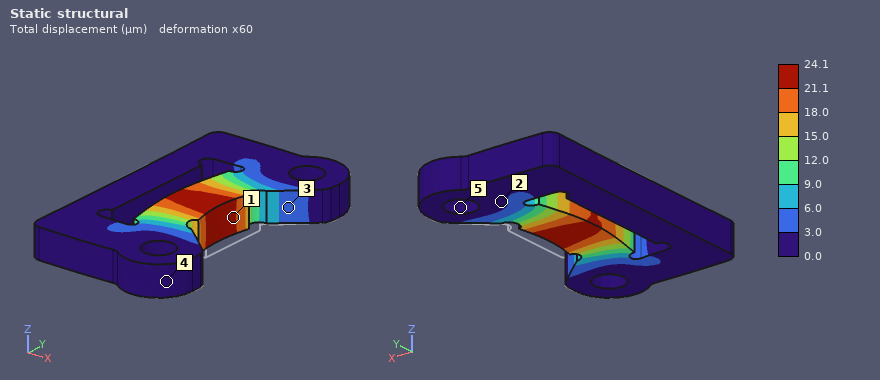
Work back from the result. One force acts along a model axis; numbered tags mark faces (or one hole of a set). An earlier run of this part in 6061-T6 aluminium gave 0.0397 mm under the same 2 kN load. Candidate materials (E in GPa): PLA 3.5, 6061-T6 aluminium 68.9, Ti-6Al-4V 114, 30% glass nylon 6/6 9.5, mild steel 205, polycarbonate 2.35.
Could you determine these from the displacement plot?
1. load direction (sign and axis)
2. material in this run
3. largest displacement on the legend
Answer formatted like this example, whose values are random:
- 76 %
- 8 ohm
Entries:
- -X
- Ti-6Al-4V
- 24.1 µm
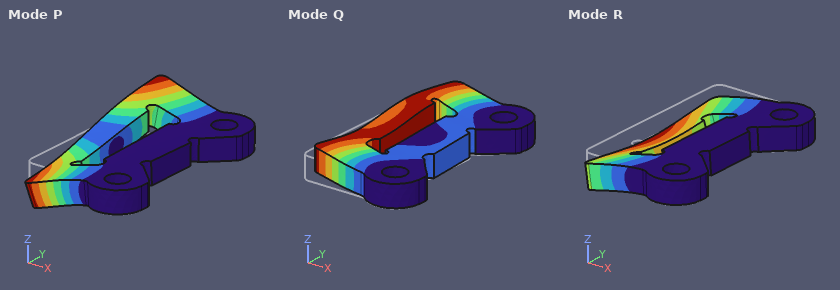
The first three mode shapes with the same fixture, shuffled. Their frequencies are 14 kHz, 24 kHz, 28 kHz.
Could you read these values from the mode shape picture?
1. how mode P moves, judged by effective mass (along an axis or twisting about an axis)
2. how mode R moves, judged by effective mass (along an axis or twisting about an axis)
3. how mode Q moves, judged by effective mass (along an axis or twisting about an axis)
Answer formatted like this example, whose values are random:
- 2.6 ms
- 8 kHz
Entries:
- twisting about X
- along Z
- along Y
